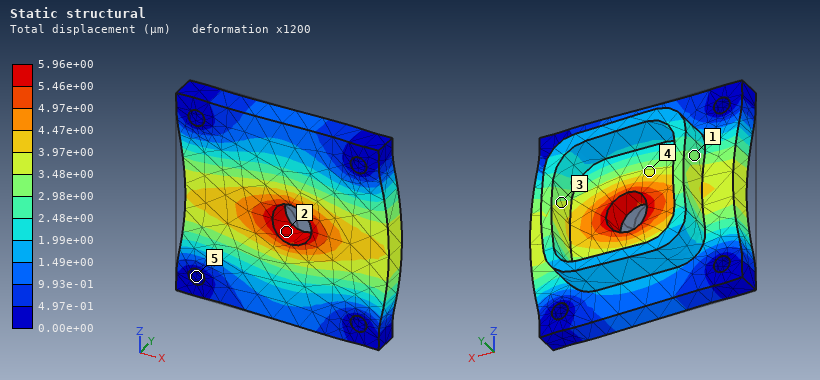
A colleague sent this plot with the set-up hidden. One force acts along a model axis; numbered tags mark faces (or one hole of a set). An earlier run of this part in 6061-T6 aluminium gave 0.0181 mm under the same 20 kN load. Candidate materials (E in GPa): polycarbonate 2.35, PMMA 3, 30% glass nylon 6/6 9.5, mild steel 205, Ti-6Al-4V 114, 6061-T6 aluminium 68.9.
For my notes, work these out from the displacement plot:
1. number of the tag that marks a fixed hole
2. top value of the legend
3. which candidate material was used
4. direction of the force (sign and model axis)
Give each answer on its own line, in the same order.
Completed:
5
5.96e+00 µm
mild steel
+X
